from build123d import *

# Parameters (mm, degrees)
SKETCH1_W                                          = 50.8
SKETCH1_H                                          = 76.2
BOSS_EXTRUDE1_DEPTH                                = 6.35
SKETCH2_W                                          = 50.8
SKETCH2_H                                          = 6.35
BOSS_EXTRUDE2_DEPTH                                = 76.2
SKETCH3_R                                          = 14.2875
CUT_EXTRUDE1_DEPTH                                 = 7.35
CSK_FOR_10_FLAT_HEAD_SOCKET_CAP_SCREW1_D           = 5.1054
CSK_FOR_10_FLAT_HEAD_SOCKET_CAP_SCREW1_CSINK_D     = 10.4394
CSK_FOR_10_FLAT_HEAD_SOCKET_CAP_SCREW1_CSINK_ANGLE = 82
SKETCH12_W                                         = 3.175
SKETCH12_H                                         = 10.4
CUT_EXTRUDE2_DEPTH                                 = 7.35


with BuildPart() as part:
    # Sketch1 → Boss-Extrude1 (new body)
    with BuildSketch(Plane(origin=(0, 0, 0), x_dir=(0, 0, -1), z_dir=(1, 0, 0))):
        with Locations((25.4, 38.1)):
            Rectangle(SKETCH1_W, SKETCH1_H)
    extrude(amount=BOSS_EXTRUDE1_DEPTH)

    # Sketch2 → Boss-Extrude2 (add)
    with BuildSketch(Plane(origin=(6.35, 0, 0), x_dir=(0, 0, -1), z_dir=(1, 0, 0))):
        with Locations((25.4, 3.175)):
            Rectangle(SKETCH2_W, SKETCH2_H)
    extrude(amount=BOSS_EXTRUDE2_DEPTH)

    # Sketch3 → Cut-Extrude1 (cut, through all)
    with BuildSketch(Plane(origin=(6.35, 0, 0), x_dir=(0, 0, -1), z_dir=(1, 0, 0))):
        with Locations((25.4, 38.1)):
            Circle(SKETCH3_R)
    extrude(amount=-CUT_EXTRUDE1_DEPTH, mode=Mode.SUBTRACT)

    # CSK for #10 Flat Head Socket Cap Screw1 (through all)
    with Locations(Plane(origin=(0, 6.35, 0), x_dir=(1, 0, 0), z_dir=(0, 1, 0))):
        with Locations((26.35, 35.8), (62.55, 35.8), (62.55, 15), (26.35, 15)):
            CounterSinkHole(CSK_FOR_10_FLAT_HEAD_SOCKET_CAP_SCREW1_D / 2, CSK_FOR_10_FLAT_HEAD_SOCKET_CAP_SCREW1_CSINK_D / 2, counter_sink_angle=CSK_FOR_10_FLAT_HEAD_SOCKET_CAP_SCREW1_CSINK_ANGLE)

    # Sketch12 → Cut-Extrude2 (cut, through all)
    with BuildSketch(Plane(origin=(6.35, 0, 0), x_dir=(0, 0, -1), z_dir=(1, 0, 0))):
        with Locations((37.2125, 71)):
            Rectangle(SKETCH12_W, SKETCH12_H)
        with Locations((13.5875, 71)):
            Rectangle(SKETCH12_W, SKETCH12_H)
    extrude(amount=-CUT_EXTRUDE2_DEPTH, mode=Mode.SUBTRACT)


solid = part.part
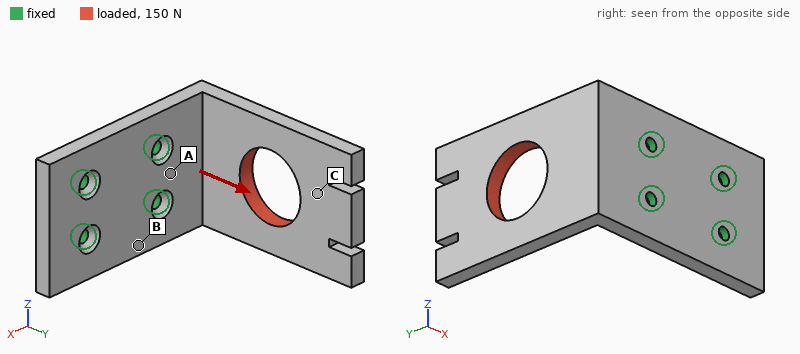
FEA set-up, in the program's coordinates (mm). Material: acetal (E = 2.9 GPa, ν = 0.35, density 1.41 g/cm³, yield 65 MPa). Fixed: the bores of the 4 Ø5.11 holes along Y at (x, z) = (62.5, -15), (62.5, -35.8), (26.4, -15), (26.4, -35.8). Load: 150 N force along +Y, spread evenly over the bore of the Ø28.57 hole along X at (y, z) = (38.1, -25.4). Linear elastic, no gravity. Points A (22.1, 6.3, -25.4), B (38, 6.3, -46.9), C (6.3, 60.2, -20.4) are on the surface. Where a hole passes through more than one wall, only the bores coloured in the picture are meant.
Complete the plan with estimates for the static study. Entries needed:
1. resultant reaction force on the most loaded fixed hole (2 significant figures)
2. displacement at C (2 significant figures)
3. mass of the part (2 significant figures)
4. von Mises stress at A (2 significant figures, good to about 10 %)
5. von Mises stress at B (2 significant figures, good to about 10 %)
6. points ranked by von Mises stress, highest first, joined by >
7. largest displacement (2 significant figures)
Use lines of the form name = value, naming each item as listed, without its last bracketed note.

resultant reaction force on the most loaded fixed hole = 120 N
displacement at C = 1.0 mm
mass of the part = 62 g
von Mises stress at A = 8.6 MPa
von Mises stress at B = 2.9 MPa
points ranked by von Mises stress, highest first, joined by > = A > B > C
largest displacement = 1.3 mm
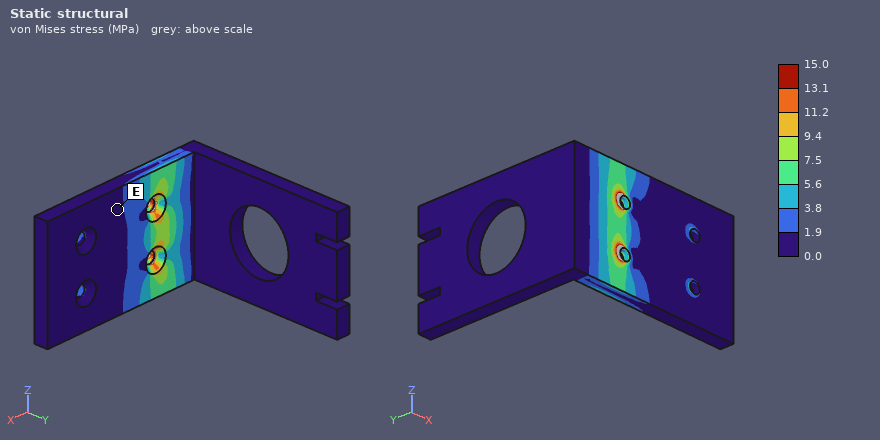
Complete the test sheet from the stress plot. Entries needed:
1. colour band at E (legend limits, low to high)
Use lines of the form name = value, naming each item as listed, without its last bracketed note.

colour band at E = 0.0 to 1.9 MPa
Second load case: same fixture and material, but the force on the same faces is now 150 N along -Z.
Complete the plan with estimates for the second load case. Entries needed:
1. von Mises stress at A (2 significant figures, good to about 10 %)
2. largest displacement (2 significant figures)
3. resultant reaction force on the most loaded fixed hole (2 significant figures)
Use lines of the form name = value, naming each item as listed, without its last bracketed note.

von Mises stress at A = 7.9 MPa
largest displacement = 1.3 mm
resultant reaction force on the most loaded fixed hole = 280 N
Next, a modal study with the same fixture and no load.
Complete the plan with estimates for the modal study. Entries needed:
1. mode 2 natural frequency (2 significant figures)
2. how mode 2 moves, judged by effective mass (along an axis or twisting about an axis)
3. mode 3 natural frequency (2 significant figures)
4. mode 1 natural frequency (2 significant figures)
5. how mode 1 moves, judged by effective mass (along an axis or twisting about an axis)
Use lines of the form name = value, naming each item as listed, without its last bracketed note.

mode 2 natural frequency = 370 Hz
how mode 2 moves, judged by effective mass = along Z
mode 3 natural frequency = 700 Hz
mode 1 natural frequency = 180 Hz
how mode 1 moves, judged by effective mass = along X
